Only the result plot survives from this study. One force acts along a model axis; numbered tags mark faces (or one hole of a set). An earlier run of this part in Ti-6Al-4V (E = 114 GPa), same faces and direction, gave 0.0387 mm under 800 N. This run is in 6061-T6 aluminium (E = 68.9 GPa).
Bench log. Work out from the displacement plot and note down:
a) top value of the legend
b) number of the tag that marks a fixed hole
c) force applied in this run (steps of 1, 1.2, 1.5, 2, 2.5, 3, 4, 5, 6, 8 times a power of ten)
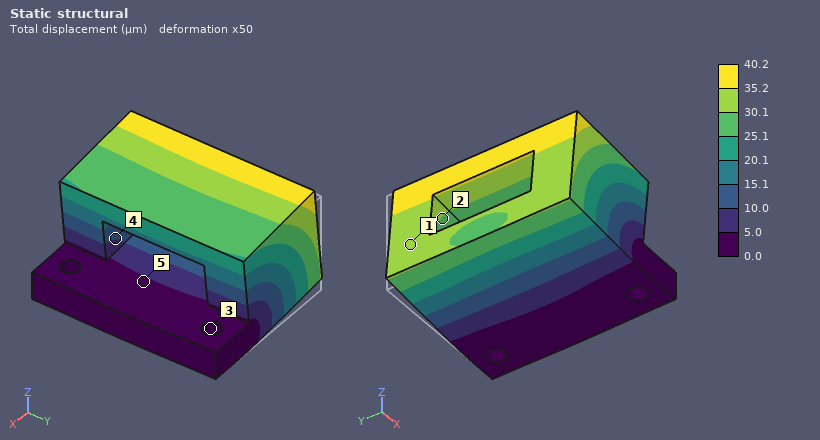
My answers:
40.2 µm
3
500 N
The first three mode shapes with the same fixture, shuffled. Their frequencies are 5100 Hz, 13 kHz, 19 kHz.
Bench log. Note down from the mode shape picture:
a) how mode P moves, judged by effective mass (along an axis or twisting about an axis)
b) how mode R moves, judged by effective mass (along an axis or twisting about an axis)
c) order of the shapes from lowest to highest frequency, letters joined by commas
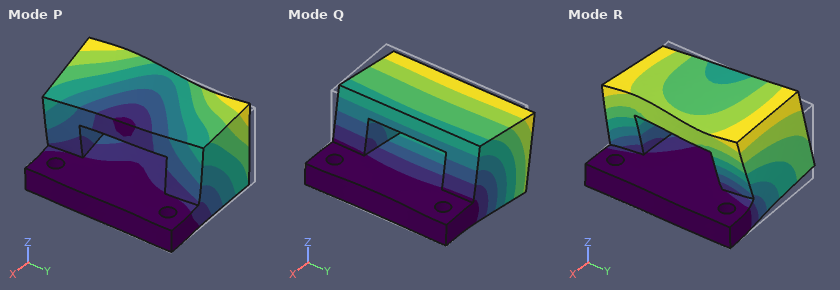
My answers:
along Y
along Y
Q, R, P
